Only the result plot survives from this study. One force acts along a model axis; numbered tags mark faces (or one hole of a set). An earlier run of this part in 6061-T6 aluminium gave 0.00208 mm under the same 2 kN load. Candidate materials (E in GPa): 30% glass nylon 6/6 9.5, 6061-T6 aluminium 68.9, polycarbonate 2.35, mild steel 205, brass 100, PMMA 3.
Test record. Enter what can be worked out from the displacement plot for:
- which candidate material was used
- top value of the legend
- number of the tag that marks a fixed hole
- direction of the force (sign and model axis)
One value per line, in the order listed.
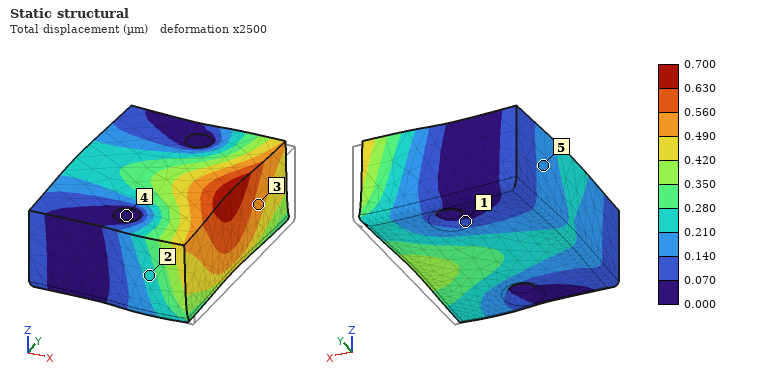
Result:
mild steel
0.700 µm
4
-X
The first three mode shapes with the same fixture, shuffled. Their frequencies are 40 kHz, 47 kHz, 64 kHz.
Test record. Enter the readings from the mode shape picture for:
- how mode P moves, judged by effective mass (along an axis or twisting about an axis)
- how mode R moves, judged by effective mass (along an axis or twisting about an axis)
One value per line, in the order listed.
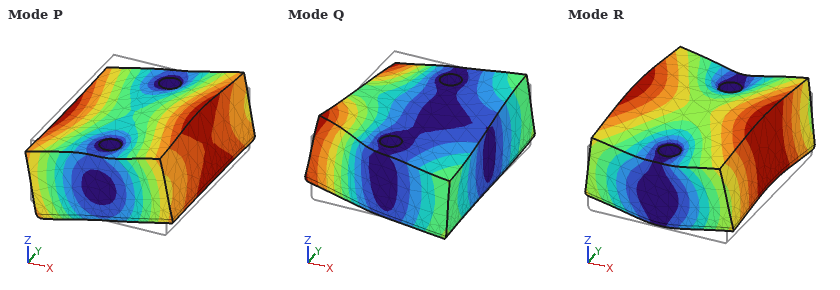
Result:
twisting about Y
along Z
